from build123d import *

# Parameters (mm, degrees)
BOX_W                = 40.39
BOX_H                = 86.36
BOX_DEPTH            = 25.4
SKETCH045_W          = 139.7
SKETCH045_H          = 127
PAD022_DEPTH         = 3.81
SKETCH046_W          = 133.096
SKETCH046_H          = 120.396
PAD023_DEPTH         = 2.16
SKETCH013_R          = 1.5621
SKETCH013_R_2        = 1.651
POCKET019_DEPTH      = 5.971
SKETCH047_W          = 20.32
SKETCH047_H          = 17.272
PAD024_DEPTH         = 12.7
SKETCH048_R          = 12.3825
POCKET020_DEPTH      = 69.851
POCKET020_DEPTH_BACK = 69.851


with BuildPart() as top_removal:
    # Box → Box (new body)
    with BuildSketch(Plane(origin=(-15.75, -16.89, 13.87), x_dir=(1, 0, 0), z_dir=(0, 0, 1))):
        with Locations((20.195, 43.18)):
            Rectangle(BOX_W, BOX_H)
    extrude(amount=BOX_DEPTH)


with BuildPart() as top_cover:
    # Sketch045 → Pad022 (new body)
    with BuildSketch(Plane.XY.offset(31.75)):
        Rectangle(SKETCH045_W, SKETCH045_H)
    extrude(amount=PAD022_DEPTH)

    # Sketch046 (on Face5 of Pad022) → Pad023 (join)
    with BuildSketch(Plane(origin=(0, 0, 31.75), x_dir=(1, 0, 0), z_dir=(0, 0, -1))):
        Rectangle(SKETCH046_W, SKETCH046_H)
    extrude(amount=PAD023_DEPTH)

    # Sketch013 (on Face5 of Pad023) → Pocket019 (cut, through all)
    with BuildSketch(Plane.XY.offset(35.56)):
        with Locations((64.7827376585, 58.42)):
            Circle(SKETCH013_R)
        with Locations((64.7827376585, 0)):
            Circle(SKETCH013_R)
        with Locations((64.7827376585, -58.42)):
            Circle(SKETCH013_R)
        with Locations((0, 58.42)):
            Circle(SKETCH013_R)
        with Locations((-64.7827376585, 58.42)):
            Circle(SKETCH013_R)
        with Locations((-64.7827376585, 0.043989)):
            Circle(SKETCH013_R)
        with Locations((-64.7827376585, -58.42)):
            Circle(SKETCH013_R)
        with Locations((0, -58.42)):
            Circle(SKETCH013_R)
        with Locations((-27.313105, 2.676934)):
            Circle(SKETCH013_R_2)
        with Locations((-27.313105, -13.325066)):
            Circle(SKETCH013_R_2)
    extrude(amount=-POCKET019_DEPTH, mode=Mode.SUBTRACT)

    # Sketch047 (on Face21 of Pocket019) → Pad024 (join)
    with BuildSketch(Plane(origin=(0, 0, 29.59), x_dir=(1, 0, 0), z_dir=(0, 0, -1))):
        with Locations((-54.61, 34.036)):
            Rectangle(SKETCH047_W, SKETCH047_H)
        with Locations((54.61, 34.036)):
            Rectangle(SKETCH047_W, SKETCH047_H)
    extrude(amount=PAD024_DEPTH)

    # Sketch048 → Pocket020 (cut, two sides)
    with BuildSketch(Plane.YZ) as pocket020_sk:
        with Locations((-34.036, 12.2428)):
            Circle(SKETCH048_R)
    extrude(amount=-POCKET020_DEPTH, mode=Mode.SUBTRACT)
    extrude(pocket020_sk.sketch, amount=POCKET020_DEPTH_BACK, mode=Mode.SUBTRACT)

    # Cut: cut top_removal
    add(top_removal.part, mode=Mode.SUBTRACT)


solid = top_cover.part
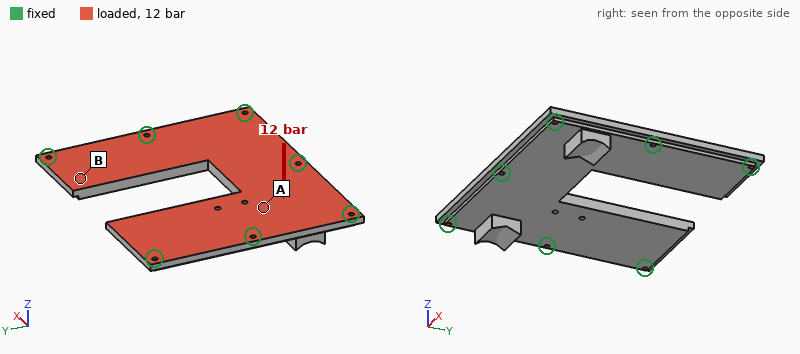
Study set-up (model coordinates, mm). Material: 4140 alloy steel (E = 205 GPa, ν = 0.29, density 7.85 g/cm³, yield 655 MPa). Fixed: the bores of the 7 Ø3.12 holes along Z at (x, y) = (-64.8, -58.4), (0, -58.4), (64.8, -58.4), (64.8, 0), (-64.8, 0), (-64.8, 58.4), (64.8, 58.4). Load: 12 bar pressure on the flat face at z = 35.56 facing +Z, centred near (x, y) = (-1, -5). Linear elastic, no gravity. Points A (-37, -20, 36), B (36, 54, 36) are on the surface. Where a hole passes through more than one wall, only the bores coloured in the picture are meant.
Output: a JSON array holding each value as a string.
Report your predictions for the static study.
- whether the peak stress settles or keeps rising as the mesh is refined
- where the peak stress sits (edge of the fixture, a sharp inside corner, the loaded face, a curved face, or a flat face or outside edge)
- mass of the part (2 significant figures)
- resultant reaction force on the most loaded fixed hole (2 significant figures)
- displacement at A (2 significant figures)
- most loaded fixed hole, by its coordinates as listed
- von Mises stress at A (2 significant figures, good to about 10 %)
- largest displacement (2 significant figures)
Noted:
["keeps rising", "edge of the fixture", "680 g", "4.3 kN", "0.11 mm", "(0, -58.4)", "98 MPa", "0.39 mm"]
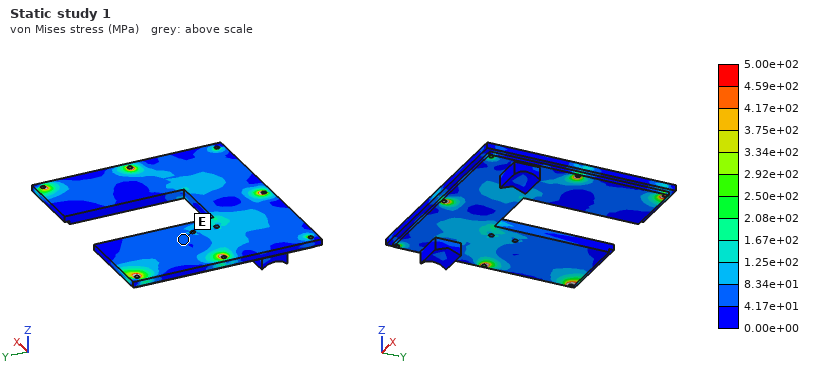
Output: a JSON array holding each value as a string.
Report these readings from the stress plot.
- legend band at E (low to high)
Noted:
["4.17e+01 to 8.34e+01 MPa"]
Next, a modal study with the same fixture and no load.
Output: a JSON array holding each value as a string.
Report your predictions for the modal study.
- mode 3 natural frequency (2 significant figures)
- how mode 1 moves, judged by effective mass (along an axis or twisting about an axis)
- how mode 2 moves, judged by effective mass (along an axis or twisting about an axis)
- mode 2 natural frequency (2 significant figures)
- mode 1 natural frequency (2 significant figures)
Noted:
["3400 Hz", "along Z", "along Z", "2400 Hz", "1800 Hz"]
